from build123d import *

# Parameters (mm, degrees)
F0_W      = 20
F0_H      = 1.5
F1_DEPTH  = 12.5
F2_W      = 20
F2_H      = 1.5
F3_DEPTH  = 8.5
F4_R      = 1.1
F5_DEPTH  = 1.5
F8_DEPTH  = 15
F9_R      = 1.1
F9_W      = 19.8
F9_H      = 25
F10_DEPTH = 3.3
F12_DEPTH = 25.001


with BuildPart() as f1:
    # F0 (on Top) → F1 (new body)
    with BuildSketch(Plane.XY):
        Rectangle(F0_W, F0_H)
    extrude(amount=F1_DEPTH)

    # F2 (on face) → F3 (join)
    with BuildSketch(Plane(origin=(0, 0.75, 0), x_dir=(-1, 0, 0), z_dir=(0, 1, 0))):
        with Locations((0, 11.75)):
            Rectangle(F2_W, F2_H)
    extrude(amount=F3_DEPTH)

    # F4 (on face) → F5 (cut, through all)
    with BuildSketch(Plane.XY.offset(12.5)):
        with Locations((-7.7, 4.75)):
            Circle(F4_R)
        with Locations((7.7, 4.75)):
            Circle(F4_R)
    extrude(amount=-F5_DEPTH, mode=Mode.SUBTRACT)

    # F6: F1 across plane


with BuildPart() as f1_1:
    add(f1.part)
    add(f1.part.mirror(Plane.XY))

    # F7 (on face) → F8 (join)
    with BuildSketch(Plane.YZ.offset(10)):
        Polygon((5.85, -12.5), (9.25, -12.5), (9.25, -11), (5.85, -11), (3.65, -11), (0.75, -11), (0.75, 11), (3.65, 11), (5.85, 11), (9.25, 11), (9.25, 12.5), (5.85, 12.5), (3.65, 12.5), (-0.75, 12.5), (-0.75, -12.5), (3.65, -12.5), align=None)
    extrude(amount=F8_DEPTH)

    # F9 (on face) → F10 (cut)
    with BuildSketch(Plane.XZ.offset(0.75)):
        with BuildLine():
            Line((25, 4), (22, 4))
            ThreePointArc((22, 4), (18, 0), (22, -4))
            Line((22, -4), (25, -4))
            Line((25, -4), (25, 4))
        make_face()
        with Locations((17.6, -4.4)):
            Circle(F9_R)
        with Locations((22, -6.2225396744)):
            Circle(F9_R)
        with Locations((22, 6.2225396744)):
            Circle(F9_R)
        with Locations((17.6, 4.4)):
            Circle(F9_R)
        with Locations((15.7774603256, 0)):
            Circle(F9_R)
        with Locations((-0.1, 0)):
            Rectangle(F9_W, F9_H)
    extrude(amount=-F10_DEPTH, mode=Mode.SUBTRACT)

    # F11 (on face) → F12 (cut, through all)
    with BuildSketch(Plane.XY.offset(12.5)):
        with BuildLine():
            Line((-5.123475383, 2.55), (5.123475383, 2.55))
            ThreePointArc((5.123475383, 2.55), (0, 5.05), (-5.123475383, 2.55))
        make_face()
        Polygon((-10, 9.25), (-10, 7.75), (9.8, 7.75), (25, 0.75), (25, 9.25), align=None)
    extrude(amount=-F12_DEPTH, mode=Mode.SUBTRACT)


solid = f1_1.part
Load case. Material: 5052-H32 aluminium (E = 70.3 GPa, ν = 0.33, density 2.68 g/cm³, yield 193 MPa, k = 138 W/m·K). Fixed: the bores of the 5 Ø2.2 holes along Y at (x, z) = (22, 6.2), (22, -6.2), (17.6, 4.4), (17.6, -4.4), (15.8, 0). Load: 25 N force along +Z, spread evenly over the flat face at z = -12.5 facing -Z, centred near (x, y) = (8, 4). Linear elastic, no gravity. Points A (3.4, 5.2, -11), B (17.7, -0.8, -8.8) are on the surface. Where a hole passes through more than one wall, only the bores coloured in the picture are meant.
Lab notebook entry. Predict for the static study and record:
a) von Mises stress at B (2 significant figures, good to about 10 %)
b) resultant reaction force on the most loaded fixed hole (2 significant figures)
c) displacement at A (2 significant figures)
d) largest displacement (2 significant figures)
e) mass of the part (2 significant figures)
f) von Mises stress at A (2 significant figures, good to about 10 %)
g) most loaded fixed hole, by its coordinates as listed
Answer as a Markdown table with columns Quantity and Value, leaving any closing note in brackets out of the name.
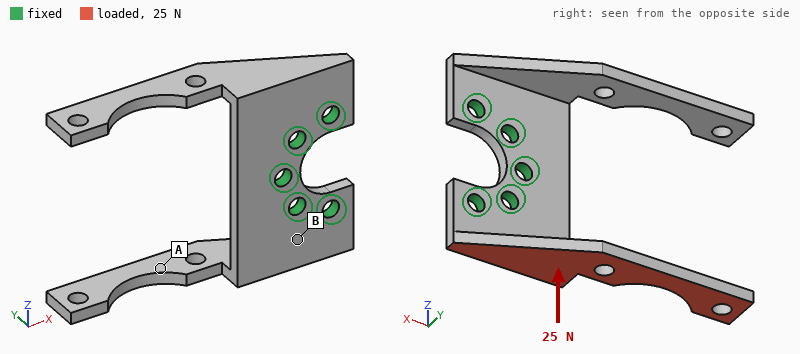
| Quantity | Value |
|---|---|
| von Mises stress at B | 17 MPa |
| resultant reaction force on the most loaded fixed hole | 22 N |
| displacement at A | 0.10 mm |
| largest displacement | 0.36 mm |
| mass of the part | 2.3 g |
| von Mises stress at A | 48 MPa |
| most loaded fixed hole, by its coordinates as listed | (15.8, 0) |
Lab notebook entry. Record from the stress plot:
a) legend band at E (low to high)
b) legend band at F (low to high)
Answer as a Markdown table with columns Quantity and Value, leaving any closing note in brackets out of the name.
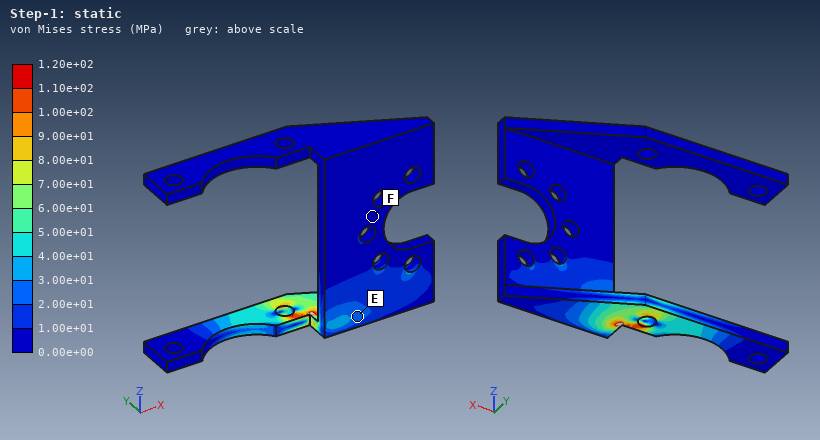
| Quantity | Value |
|---|---|
| legend band at E | 2.00e+01 to 3.00e+01 MPa |
| legend band at F | 0.00e+00 to 1.00e+01 MPa |
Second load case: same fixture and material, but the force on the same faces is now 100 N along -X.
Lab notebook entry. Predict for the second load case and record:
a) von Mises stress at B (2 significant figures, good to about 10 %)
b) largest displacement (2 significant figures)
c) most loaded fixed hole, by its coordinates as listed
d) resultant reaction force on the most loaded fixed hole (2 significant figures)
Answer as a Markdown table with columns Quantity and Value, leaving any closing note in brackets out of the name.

| Quantity | Value |
|---|---|
| von Mises stress at B | 25 MPa |
| largest displacement | 0.14 mm |
| most loaded fixed hole, by its coordinates as listed | (22, -6.2) |
| resultant reaction force on the most loaded fixed hole | 110 N |
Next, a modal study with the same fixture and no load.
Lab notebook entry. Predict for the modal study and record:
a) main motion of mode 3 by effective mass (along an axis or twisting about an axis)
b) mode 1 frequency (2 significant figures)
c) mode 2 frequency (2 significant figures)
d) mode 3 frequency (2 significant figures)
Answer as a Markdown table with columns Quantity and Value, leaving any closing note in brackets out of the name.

| Quantity | Value |
|---|---|
| main motion of mode 3 by effective mass | twisting about X |
| mode 1 frequency | 2100 Hz |
| mode 2 frequency | 2100 Hz |
| mode 3 frequency | 3500 Hz |
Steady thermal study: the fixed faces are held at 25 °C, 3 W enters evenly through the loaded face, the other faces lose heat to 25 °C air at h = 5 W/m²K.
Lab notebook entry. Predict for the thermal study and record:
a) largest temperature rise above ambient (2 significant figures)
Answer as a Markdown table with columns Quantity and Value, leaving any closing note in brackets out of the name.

| Quantity | Value |
|---|---|
| largest temperature rise above ambient | 38 K |
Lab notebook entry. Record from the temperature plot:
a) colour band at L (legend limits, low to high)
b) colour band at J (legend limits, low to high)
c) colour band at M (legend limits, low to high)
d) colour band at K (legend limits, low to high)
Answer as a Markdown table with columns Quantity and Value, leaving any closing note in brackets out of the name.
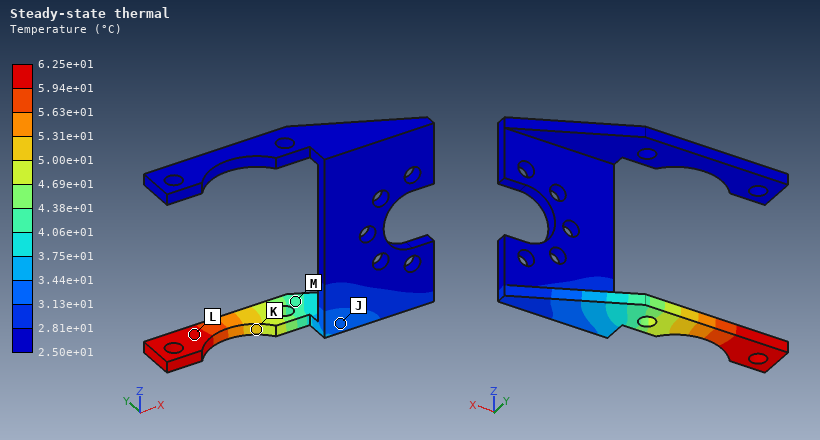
| Quantity | Value |
|---|---|
| colour band at L | 5.94e+01 to 6.25e+01 °C |
| colour band at J | 3.13e+01 to 3.44e+01 °C |
| colour band at M | 4.06e+01 to 4.38e+01 °C |
| colour band at K | 5.00e+01 to 5.31e+01 °C |
